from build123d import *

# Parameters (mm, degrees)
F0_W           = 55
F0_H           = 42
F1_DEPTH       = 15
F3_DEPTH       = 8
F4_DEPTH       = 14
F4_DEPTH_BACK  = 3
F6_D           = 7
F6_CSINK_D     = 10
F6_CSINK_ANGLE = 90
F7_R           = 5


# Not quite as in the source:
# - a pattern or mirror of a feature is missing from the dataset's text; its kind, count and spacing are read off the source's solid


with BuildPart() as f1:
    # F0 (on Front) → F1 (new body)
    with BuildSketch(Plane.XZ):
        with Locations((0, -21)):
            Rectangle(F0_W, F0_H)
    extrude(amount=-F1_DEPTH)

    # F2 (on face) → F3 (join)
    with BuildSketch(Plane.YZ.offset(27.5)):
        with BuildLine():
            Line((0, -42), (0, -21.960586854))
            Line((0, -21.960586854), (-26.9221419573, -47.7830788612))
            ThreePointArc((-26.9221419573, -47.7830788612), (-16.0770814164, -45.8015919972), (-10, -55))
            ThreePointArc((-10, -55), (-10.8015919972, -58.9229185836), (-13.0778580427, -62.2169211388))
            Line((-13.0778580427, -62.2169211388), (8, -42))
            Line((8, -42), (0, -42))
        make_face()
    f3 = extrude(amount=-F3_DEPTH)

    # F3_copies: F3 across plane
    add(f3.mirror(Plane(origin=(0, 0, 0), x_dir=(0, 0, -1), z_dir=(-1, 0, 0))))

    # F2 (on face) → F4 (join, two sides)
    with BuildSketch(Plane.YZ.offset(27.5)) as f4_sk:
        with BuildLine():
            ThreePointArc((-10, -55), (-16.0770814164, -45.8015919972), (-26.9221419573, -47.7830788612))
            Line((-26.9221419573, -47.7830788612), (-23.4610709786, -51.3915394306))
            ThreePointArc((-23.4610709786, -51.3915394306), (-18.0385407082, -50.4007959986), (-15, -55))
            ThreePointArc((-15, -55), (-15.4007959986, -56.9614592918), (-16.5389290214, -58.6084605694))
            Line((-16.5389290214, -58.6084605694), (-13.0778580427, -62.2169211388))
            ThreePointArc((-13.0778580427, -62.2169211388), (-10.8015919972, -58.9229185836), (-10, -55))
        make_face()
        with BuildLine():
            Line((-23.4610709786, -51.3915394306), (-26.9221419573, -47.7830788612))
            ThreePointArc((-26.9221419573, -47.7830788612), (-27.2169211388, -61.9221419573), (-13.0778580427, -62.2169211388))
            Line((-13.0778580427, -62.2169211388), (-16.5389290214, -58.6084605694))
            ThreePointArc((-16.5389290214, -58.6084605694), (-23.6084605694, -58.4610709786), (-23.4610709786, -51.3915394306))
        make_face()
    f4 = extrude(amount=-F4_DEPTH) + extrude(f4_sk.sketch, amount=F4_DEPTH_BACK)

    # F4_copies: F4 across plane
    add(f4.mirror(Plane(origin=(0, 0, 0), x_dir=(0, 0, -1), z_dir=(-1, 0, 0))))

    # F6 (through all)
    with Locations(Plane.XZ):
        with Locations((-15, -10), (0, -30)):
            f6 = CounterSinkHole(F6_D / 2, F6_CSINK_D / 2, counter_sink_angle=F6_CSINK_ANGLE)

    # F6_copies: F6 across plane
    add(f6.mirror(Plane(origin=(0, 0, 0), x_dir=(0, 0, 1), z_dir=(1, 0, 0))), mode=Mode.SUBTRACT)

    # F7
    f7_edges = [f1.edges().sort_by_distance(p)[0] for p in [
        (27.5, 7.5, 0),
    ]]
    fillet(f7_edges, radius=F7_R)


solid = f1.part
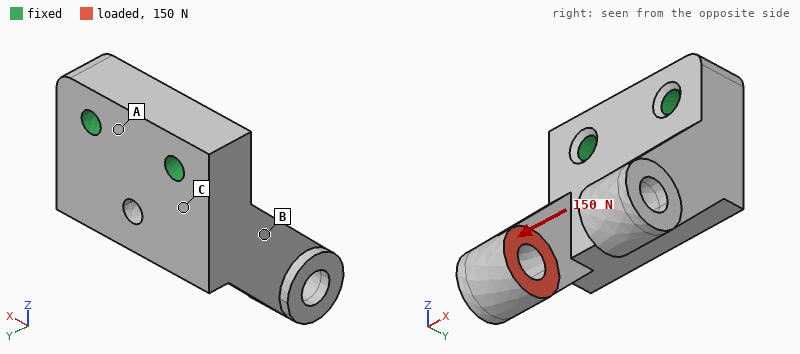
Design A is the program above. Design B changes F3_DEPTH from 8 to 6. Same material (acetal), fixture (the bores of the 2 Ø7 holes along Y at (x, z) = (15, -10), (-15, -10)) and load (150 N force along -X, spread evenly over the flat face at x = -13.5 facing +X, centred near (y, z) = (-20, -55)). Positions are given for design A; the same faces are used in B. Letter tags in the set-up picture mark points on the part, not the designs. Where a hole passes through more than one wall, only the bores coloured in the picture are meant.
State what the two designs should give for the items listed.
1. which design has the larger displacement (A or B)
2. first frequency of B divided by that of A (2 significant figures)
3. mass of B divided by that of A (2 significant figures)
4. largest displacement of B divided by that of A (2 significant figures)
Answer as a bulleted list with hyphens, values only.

- B
- 0.75
- 0.96
- 1.9
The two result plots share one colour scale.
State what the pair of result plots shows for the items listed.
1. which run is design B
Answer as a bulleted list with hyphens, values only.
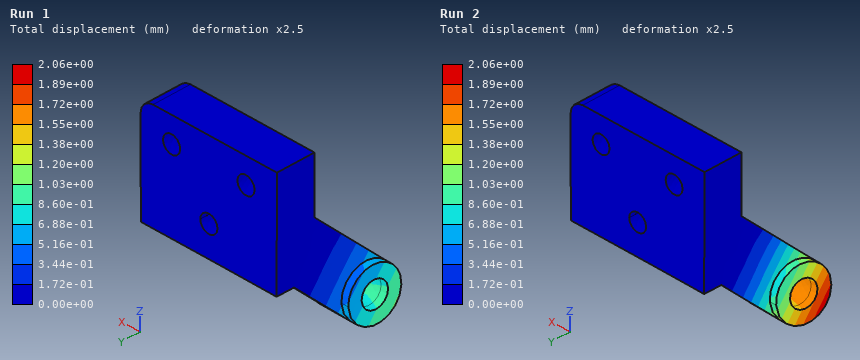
- Run 2
